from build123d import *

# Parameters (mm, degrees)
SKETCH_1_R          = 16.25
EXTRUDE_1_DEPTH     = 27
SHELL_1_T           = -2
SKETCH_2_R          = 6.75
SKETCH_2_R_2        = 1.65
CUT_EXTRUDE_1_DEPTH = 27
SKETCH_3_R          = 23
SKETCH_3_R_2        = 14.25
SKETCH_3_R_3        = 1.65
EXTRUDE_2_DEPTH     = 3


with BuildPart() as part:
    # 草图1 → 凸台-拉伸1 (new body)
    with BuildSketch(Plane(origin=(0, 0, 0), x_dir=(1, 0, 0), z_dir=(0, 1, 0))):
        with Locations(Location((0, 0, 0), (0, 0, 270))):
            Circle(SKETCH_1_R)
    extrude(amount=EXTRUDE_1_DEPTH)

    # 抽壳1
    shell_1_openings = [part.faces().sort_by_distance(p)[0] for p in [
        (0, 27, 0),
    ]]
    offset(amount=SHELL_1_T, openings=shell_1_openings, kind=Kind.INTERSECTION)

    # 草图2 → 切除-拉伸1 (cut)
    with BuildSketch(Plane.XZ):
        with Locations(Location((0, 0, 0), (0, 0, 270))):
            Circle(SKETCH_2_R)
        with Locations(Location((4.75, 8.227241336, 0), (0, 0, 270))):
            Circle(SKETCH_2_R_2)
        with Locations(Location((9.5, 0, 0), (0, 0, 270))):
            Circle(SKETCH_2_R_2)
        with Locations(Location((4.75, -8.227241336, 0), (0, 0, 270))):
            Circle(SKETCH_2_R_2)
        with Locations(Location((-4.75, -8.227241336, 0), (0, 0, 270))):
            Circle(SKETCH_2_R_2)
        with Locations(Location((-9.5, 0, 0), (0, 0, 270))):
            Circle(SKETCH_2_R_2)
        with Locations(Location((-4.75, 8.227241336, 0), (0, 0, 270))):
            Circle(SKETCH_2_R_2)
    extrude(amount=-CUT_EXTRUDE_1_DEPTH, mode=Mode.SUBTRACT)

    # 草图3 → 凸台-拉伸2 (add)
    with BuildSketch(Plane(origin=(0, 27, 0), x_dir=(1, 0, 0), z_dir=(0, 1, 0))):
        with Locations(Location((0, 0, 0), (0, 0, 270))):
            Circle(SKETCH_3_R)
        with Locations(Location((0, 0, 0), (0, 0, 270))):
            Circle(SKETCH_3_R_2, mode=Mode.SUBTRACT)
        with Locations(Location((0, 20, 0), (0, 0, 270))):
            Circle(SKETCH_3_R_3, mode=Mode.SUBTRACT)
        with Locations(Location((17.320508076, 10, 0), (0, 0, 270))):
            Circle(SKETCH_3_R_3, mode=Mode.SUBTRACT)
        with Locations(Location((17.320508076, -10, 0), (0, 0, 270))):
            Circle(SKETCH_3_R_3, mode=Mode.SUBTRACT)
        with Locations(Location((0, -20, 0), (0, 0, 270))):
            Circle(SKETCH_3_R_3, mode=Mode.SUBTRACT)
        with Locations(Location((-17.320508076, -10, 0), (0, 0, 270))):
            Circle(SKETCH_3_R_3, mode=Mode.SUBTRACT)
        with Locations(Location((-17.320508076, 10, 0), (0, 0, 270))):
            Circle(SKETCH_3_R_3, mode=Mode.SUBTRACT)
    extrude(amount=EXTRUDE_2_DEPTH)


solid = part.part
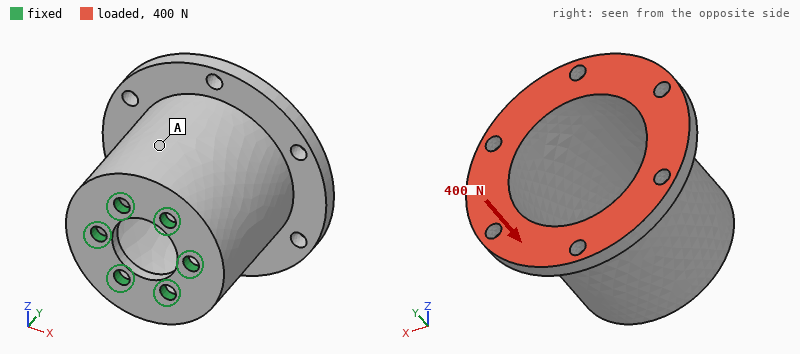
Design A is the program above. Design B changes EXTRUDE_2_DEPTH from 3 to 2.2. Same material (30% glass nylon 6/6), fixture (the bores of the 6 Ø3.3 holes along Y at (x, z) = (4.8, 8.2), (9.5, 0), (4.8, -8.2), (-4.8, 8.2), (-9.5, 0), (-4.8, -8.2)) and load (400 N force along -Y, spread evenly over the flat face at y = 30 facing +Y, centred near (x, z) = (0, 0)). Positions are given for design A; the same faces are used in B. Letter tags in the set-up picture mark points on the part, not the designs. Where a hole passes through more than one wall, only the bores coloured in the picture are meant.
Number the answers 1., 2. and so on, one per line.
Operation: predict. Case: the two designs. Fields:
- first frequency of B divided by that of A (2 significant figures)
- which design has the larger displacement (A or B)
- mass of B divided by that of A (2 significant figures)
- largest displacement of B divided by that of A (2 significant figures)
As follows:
1. 1.1
2. B
3. 0.91
4. 1.3
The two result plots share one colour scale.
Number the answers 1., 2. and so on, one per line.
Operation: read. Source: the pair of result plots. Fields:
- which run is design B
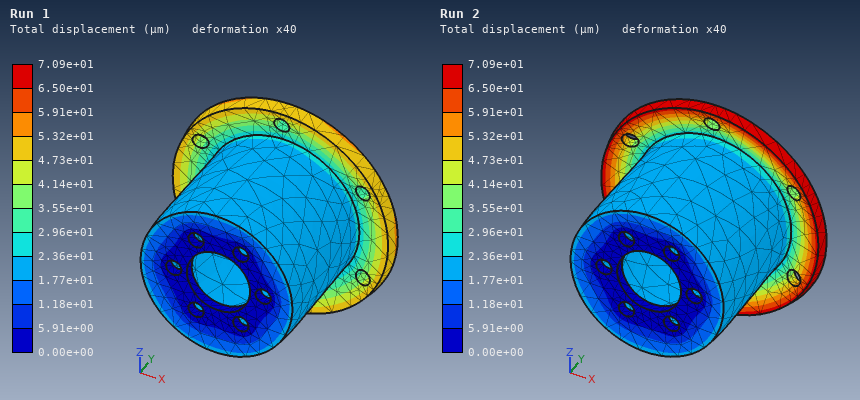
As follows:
1. Run 2
